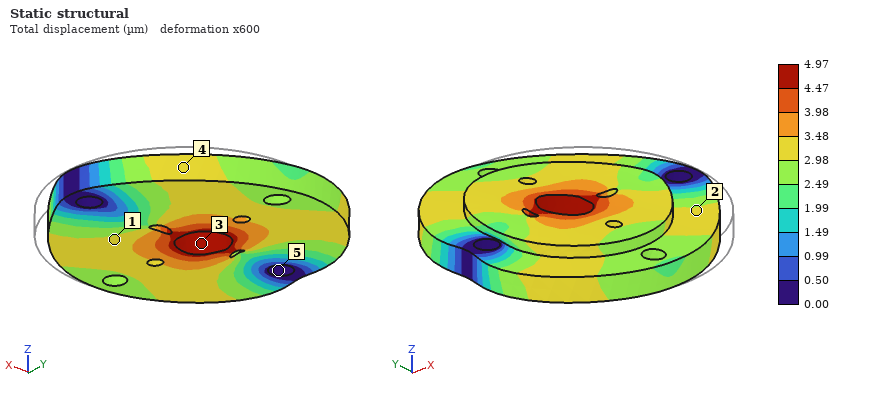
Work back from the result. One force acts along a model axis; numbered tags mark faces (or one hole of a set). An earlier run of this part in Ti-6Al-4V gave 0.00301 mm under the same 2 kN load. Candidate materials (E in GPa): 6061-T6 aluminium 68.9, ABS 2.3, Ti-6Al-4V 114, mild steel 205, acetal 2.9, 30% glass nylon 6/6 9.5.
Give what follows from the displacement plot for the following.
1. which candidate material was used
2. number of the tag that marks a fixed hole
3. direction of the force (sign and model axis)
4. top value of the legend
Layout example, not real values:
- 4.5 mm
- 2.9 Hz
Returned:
- 6061-T6 aluminium
- 5
- -X
- 4.97 µm
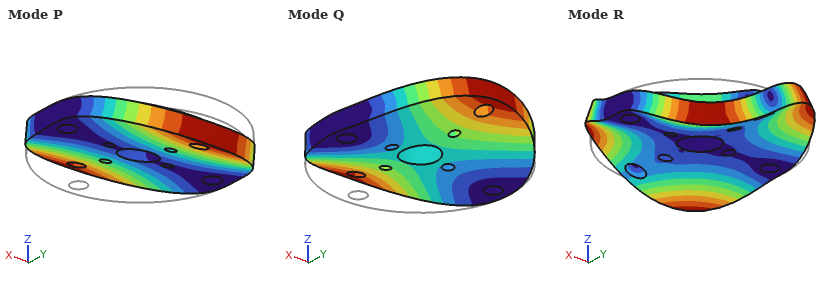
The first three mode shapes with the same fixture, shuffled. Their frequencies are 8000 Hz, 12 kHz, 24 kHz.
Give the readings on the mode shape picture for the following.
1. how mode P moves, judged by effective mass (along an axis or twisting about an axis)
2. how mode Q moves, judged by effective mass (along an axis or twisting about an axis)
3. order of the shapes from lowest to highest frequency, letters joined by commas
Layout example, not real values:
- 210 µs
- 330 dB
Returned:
- twisting about X
- along Z
- P, Q, R
